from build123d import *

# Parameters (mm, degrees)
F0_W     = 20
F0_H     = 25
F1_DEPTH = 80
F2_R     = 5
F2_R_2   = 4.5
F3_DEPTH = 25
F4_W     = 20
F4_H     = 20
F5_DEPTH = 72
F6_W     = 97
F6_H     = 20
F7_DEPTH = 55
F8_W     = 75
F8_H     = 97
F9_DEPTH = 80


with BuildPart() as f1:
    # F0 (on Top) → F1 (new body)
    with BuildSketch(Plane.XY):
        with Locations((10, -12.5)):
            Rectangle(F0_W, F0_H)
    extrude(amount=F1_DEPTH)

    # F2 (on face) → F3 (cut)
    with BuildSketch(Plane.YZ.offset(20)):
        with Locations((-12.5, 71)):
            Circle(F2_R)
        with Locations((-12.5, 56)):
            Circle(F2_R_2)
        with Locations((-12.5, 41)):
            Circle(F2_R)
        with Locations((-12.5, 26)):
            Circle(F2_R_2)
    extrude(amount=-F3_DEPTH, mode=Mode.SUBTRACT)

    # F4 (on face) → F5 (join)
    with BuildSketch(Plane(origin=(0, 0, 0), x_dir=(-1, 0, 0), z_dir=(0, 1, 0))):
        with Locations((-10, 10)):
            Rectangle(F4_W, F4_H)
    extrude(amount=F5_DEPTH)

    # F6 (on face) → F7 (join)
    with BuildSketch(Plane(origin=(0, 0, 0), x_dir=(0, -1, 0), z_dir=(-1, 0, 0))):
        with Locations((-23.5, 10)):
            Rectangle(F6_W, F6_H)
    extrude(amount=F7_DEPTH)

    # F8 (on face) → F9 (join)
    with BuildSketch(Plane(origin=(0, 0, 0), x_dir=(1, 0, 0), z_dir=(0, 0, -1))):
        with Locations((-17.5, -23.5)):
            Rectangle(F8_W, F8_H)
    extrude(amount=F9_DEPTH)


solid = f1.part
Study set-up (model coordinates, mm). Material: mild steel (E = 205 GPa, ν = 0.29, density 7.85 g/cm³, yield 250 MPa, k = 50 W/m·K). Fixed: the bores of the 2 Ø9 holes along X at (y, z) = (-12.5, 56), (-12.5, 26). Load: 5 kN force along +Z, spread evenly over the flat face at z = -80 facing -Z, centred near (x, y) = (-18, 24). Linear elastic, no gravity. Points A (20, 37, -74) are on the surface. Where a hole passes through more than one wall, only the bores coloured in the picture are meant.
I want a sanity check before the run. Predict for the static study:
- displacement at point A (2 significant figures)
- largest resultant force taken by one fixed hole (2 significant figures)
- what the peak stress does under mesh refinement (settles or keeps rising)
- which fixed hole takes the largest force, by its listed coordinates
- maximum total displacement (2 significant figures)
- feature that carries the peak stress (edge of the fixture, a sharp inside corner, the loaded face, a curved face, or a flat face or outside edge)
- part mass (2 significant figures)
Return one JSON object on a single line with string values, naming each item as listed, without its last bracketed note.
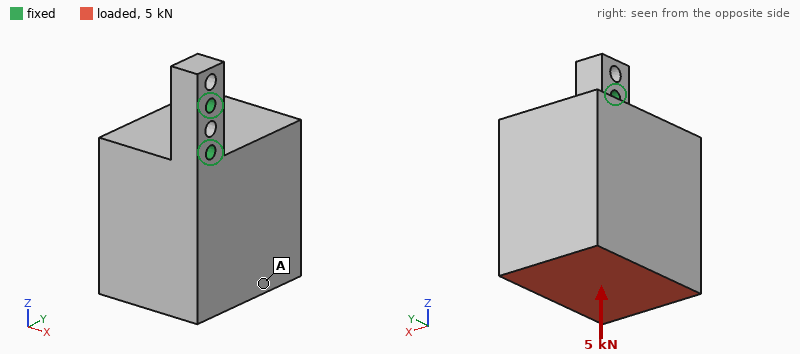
{"displacement at point A": "0.095 mm", "largest resultant force taken by one fixed hole": "5.0 kN", "what the peak stress does under mesh refinement": "keeps rising", "which fixed hole takes the largest force, by its listed coordinates": "(-12.5, 26)", "maximum total displacement": "0.14 mm", "feature that carries the peak stress": "edge of the fixture", "part mass": "5.9 kg"}
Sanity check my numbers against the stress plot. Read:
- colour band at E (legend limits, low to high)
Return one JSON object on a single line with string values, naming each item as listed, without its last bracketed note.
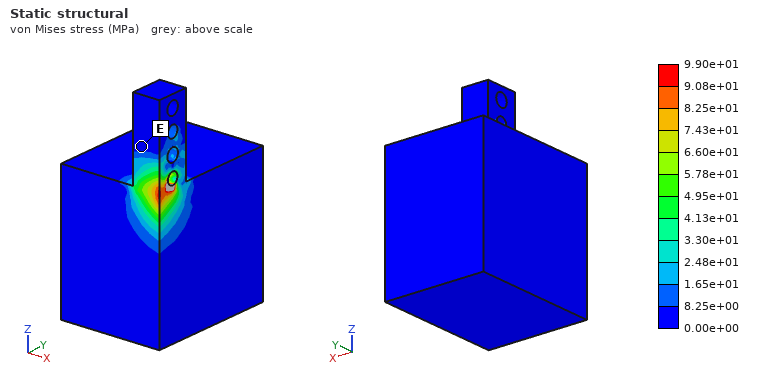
{"colour band at E": "0.00e+00 to 8.25e+00 MPa"}
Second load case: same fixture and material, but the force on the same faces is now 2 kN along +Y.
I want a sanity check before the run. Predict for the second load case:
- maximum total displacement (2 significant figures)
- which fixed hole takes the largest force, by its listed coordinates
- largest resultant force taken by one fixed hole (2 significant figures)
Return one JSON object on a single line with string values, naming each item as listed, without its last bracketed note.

{"maximum total displacement": "0.12 mm", "which fixed hole takes the largest force, by its listed coordinates": "(-12.5, 26)", "largest resultant force taken by one fixed hole": "4.1 kN"}
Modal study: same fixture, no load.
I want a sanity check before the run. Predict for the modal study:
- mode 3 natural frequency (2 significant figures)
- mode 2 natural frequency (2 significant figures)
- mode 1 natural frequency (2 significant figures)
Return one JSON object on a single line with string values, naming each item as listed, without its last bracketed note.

{"mode 3 natural frequency": "860 Hz", "mode 2 natural frequency": "440 Hz", "mode 1 natural frequency": "410 Hz"}
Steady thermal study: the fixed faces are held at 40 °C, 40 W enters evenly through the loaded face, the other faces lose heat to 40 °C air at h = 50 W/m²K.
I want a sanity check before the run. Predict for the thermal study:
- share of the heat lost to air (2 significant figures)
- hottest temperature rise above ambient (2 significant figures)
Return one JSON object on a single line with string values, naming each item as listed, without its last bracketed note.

{"share of the heat lost to air": "65 %", "hottest temperature rise above ambient": "18 K"}
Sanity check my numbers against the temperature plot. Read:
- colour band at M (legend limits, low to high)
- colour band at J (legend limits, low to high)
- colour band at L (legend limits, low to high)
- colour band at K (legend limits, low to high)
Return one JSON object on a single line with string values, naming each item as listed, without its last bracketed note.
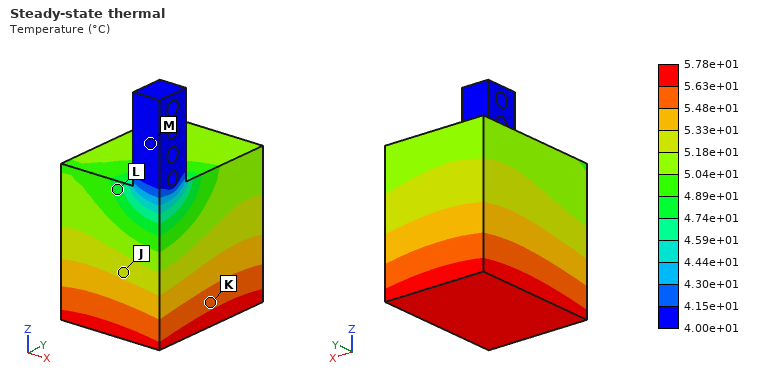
{"colour band at M": "4.00e+01 to 4.15e+01 °C", "colour band at J": "5.18e+01 to 5.33e+01 °C", "colour band at L": "4.74e+01 to 4.89e+01 °C", "colour band at K": "5.48e+01 to 5.63e+01 °C"}
